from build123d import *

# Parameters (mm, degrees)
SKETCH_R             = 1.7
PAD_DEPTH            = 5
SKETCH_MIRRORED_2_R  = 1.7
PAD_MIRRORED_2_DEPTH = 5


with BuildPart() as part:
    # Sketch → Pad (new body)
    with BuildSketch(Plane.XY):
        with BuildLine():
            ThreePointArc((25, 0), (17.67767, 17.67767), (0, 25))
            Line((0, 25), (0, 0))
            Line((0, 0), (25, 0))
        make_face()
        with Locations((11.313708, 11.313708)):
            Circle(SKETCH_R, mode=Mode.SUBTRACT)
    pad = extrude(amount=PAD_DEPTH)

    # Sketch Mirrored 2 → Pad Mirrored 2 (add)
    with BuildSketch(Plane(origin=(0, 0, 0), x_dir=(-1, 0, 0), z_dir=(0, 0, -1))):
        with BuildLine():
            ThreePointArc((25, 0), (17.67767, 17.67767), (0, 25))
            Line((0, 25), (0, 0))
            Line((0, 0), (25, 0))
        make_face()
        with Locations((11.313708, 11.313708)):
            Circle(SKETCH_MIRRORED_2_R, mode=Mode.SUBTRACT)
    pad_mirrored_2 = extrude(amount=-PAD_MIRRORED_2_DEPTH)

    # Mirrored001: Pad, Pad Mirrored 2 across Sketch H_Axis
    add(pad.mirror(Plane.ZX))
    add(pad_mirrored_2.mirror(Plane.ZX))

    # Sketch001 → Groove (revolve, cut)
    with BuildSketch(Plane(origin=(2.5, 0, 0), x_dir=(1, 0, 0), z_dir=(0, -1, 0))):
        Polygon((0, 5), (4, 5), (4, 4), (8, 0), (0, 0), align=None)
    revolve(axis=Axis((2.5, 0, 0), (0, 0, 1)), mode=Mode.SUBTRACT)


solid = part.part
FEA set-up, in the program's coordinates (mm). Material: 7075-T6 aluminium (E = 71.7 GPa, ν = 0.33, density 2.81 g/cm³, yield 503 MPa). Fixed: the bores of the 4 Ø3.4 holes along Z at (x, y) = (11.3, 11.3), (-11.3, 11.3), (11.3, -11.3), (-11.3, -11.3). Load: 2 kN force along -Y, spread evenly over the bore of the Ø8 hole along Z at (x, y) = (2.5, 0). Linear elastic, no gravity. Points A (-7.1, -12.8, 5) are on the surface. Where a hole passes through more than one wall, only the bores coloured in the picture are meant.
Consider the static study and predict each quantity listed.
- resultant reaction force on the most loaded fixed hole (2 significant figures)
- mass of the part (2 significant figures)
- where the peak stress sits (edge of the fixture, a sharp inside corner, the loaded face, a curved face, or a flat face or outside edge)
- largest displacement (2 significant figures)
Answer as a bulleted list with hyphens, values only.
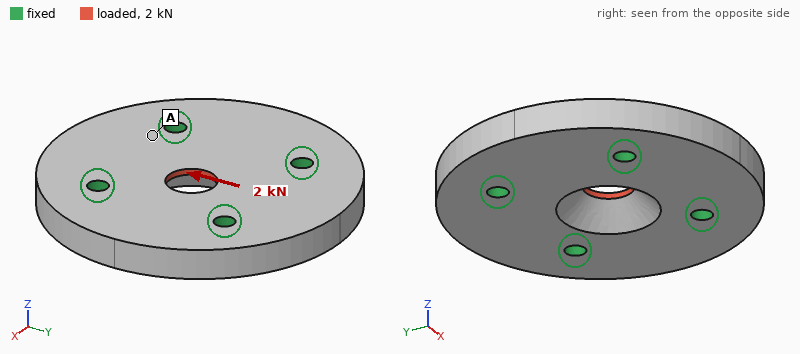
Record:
- 600 N
- 26 g
- the loaded face
- 7.5 µm
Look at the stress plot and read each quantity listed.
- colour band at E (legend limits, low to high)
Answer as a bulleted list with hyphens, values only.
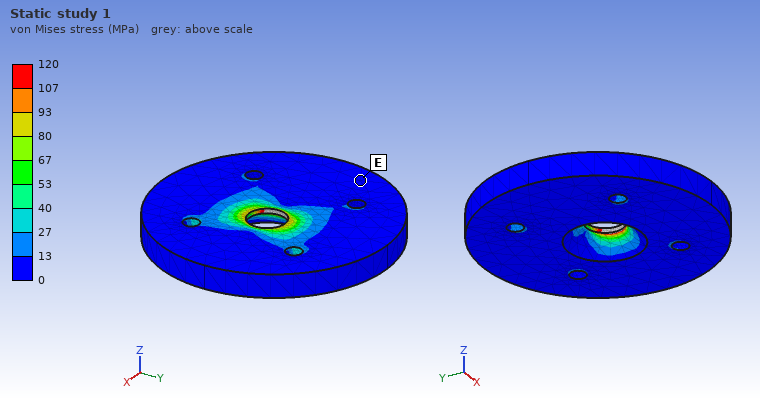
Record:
- 0 to 13 MPa
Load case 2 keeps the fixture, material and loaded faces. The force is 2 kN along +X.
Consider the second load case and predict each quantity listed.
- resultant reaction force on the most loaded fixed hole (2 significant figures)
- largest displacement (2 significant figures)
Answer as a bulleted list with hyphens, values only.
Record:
- 570 N
- 7.9 µm
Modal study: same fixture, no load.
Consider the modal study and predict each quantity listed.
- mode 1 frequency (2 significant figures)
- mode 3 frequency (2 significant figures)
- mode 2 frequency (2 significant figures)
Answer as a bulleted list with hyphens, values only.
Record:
- 19 kHz
- 21 kHz
- 21 kHz
